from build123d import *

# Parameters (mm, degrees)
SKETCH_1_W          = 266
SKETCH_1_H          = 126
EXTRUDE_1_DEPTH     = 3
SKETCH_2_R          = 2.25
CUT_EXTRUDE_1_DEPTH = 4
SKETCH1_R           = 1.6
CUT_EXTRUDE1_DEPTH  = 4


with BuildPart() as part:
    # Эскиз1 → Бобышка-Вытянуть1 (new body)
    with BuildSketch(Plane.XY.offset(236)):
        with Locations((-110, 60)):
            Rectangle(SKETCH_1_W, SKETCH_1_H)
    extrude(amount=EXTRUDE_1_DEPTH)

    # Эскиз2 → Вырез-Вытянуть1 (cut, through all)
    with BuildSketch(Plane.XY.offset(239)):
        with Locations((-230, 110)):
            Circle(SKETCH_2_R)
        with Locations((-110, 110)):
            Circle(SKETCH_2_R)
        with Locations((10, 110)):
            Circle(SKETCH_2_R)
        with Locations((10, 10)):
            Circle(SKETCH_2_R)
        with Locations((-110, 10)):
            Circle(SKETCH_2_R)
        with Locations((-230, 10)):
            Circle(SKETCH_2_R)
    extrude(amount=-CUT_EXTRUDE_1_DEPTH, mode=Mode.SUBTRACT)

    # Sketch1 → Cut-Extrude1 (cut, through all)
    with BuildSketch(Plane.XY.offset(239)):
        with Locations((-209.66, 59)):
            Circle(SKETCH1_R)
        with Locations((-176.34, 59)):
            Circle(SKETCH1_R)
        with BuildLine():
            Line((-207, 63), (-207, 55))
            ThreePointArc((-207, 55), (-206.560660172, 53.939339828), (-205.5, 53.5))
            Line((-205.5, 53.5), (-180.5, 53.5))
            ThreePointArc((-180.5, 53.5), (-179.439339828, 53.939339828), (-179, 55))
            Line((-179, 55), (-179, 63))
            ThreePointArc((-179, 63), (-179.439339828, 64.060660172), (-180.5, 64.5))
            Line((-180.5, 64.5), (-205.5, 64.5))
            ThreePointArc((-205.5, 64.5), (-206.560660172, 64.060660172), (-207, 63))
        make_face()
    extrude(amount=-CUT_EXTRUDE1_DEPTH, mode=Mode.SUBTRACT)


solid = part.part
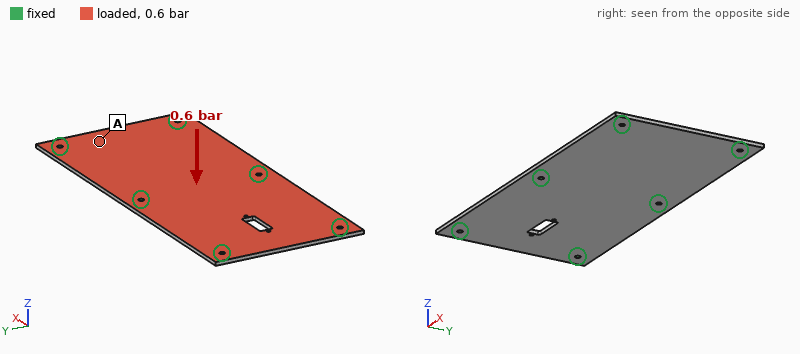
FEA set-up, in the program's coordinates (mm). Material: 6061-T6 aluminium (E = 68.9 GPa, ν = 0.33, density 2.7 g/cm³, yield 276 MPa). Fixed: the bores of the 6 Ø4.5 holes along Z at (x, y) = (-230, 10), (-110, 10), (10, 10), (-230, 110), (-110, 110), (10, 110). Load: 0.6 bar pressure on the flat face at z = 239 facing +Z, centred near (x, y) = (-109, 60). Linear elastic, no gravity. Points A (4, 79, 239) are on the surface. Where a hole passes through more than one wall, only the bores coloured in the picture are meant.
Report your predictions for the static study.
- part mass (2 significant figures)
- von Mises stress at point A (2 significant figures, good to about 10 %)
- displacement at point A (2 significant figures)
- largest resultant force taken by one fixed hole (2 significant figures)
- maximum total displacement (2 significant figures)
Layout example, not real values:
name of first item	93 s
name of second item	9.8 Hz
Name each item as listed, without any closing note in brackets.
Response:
part mass	270 g
von Mises stress at point A	16 MPa
displacement at point A	0.14 mm
largest resultant force taken by one fixed hole	470 N
maximum total displacement	0.40 mm
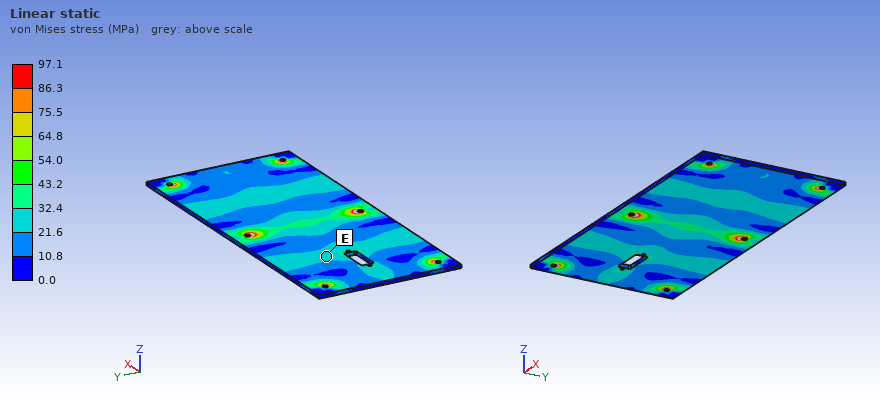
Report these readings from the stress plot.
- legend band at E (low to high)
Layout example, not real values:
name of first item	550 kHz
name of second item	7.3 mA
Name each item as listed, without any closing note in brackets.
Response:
legend band at E	21.6 to 32.4 MPa
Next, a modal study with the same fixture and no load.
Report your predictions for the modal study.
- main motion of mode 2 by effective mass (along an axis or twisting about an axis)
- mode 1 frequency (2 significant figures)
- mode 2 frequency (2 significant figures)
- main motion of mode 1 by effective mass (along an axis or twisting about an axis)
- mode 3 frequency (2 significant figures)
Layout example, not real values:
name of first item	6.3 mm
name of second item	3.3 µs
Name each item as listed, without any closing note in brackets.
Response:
main motion of mode 2 by effective mass	along Z
mode 1 frequency	810 Hz
mode 2 frequency	860 Hz
main motion of mode 1 by effective mass	twisting about Y
mode 3 frequency	1200 Hz
